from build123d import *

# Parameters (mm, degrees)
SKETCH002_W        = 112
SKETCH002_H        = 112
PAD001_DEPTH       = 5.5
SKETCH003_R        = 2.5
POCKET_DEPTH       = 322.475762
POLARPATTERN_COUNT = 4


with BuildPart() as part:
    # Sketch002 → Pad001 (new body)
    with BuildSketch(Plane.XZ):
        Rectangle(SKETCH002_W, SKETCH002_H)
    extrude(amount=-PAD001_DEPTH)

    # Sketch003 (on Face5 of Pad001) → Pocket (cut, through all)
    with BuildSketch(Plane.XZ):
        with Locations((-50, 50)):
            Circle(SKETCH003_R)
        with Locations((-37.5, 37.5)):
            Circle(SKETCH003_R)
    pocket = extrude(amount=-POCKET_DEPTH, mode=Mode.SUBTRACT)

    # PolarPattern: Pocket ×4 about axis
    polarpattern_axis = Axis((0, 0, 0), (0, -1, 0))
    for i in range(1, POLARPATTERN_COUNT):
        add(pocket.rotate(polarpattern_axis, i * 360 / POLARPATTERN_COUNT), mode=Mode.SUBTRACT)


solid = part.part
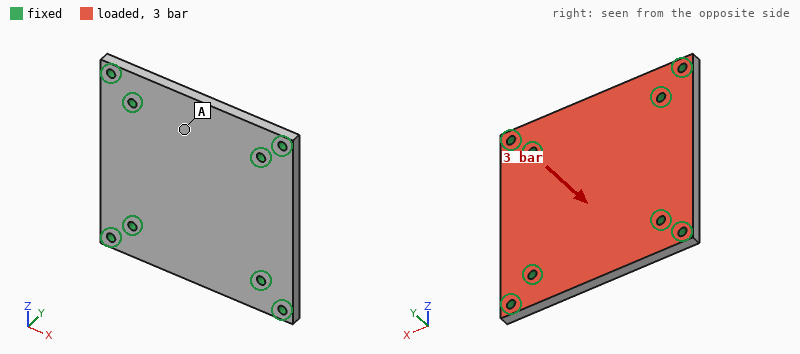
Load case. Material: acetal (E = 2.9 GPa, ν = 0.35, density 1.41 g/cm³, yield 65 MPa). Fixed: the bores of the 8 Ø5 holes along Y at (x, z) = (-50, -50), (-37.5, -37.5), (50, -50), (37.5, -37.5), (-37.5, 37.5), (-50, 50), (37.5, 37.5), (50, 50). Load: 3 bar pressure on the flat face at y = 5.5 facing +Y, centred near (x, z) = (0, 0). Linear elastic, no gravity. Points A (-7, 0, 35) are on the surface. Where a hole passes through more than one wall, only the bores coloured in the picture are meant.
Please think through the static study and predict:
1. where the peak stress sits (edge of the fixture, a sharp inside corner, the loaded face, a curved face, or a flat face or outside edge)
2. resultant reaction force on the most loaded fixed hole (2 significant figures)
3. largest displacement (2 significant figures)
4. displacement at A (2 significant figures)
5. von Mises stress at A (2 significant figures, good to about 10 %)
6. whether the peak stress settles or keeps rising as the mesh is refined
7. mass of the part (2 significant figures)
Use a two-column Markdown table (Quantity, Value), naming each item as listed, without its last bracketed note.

| Quantity | Value |
|---|---|
| where the peak stress sits | edge of the fixture |
| resultant reaction force on the most loaded fixed hole | 990 N |
| largest displacement | 1.4 mm |
| displacement at A | 0.85 mm |
| von Mises stress at A | 15 MPa |
| whether the peak stress settles or keeps rising as the mesh is refined | keeps rising |
| mass of the part | 96 g |
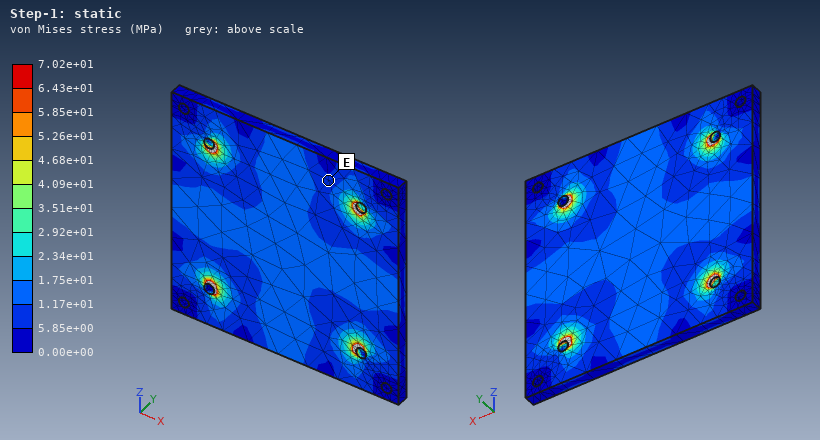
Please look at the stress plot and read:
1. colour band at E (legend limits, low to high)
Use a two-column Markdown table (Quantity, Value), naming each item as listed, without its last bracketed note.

| Quantity | Value |
|---|---|
| colour band at E | 5.85e+00 to 1.17e+01 MPa |
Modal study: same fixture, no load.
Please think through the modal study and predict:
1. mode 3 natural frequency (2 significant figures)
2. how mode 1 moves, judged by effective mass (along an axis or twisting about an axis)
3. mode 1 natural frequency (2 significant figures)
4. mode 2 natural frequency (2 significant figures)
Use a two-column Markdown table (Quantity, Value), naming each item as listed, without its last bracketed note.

| Quantity | Value |
|---|---|
| mode 3 natural frequency | 1400 Hz |
| how mode 1 moves, judged by effective mass | along Y |
| mode 1 natural frequency | 1000 Hz |
| mode 2 natural frequency | 1300 Hz |
